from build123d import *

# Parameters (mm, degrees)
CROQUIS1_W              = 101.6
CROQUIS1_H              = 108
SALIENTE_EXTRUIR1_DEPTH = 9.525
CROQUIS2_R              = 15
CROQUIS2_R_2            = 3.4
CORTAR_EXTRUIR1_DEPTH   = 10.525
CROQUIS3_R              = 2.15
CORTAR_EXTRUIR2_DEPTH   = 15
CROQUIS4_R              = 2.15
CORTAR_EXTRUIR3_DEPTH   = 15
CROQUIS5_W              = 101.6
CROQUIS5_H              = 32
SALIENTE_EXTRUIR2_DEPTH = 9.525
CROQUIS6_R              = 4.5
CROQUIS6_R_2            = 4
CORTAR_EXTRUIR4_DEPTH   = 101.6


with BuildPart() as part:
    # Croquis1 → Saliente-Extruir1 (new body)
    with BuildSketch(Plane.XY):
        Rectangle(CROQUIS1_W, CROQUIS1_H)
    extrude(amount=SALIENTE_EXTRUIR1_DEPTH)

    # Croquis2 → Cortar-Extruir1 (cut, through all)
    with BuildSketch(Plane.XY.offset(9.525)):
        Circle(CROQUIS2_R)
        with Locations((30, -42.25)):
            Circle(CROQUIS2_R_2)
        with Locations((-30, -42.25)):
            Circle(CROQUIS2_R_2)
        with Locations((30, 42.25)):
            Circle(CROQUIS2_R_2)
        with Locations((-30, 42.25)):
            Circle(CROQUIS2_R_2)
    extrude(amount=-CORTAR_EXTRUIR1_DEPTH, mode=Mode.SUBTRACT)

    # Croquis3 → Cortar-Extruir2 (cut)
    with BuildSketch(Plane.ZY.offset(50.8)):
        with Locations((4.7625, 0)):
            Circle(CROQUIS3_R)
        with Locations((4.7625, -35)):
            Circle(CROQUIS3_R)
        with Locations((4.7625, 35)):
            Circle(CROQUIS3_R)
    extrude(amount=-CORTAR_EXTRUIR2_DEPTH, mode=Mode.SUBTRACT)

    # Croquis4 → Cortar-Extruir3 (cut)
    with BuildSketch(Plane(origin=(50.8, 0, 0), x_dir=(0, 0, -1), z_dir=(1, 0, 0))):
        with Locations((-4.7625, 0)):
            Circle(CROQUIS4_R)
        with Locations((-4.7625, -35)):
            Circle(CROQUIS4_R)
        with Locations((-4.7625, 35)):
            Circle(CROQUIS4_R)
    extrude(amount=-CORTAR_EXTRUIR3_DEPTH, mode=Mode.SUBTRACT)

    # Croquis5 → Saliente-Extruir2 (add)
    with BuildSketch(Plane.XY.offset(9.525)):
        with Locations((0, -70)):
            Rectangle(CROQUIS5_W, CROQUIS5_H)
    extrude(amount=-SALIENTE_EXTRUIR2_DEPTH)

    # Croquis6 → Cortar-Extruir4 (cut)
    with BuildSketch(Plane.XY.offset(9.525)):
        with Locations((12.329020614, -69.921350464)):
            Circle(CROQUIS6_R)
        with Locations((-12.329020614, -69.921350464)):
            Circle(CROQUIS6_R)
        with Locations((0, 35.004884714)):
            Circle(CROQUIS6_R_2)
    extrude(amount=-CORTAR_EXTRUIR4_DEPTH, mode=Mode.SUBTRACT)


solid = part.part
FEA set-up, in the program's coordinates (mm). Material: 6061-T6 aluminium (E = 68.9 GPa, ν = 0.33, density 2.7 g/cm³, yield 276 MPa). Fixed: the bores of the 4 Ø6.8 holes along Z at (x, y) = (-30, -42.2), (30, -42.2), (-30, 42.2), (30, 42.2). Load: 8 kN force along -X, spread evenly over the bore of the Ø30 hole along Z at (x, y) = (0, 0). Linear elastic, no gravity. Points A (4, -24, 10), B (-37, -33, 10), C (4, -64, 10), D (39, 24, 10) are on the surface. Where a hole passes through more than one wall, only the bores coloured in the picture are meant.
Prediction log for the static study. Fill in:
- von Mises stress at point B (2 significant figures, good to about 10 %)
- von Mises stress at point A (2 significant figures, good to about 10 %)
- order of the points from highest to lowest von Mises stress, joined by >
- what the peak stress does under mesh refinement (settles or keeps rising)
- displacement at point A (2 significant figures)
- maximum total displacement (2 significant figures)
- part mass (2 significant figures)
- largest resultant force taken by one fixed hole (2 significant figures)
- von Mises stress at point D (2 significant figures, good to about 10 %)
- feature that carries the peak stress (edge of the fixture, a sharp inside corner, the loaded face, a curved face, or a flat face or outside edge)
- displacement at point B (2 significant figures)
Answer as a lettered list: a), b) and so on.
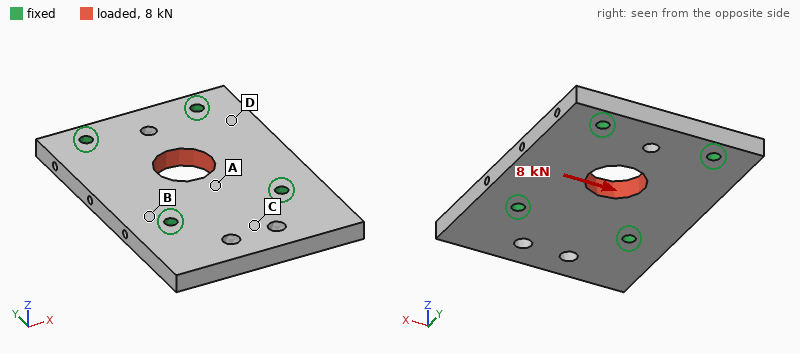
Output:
a) 7.6 MPa
b) 11 MPa
c) A > B > D > C
d) keeps rising
e) 4.8 µm
f) 9.2 µm
g) 340 g
h) 2.3 kN
i) 5.2 MPa
j) edge of the fixture
k) 2.5 µm
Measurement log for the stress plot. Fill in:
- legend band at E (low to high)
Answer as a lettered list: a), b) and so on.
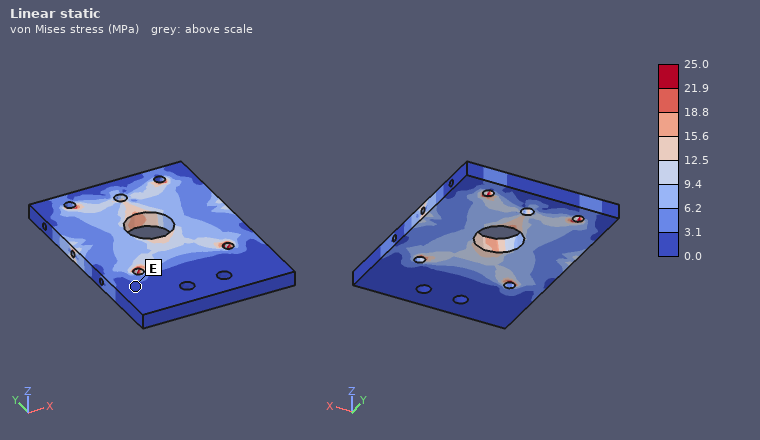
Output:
a) 0.0 to 3.1 MPa
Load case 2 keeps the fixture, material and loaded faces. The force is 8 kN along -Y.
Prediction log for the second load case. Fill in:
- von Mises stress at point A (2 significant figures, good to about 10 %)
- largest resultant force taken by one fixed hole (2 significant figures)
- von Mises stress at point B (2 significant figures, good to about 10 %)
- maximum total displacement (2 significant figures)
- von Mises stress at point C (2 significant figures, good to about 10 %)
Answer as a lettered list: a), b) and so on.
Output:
a) 7.3 MPa
b) 2.1 kN
c) 3.8 MPa
d) 6.0 µm
e) 2.3 MPa
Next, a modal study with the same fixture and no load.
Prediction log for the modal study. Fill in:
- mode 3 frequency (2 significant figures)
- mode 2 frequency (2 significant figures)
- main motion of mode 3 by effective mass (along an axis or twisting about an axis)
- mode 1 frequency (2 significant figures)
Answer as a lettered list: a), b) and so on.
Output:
a) 5900 Hz
b) 4900 Hz
c) along Z
d) 3500 Hz
